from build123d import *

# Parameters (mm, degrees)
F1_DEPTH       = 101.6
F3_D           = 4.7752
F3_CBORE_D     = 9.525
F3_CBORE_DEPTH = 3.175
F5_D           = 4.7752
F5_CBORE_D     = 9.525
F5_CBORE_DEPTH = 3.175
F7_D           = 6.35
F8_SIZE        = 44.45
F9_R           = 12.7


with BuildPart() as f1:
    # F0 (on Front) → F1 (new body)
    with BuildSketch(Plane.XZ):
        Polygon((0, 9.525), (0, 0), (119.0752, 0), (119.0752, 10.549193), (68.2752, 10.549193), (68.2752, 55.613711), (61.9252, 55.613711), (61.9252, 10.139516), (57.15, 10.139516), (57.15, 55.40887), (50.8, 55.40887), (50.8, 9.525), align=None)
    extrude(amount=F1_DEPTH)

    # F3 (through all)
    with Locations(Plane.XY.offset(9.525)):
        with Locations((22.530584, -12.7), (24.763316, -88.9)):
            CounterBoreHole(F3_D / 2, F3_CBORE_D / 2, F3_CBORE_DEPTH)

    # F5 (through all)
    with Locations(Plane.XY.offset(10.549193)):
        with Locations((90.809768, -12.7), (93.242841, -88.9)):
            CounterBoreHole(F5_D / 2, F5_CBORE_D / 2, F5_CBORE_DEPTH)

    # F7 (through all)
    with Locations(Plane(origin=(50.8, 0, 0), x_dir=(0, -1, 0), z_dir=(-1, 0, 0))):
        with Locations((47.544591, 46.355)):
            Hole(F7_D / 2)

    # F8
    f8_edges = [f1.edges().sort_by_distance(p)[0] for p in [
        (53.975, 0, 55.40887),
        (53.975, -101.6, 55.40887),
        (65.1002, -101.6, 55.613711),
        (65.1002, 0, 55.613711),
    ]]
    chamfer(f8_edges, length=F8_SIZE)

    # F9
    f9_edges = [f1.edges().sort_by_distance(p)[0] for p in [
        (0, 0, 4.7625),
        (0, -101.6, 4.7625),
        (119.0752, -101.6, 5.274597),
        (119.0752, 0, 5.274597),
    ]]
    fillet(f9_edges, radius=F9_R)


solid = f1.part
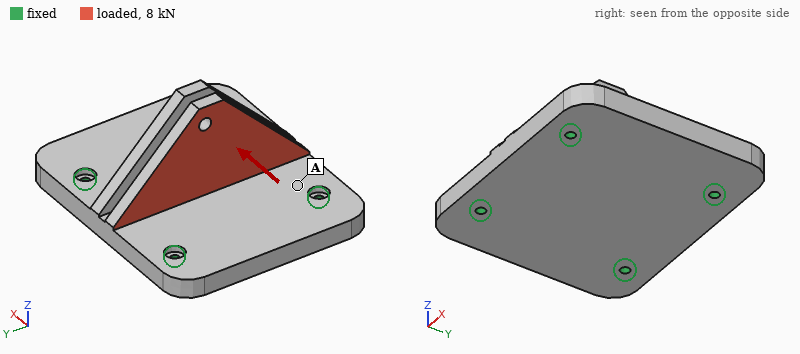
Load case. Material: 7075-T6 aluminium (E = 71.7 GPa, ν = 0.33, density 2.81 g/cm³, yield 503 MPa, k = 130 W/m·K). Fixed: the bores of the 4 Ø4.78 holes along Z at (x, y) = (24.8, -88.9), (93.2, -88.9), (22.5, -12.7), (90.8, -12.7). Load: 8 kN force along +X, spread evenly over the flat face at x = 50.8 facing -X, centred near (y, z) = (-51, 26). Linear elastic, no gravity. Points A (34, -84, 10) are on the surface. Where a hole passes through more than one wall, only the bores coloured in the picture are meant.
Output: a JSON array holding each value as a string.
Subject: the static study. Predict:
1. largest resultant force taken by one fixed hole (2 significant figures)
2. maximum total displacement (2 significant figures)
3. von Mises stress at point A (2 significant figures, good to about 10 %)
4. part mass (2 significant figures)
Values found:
["2.8 kN", "0.70 mm", "19 MPa", "430 g"]
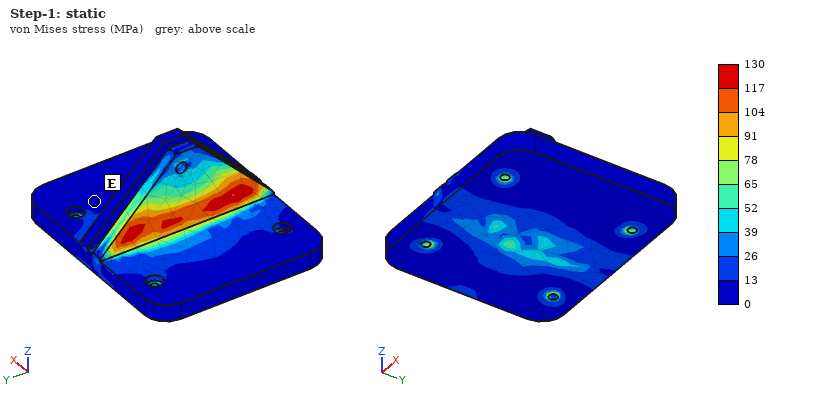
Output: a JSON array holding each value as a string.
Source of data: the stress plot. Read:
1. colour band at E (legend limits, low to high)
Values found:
["0 to 13 MPa"]
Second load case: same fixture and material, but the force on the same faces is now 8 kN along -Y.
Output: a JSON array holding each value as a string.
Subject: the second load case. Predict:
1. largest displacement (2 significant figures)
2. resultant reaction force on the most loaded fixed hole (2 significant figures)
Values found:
["63 µm", "2.8 kN"]
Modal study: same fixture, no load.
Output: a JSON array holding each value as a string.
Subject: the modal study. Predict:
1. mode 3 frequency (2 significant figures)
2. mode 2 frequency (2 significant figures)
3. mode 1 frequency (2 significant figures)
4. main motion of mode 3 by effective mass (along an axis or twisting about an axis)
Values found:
["4600 Hz", "3500 Hz", "3300 Hz", "along Z"]
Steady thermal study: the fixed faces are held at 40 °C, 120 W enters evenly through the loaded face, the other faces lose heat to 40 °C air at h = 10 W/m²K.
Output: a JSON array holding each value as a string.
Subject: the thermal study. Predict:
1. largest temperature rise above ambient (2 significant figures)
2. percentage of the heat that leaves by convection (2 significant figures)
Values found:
["65 K", "4.7 %"]
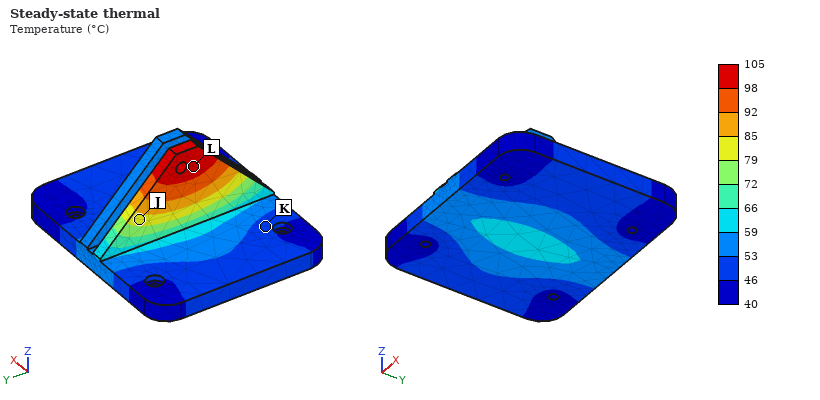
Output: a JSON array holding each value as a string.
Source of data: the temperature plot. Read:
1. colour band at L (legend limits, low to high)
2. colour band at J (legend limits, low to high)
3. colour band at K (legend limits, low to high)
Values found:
["98 to 105 °C", "79 to 85 °C", "46 to 53 °C"]
